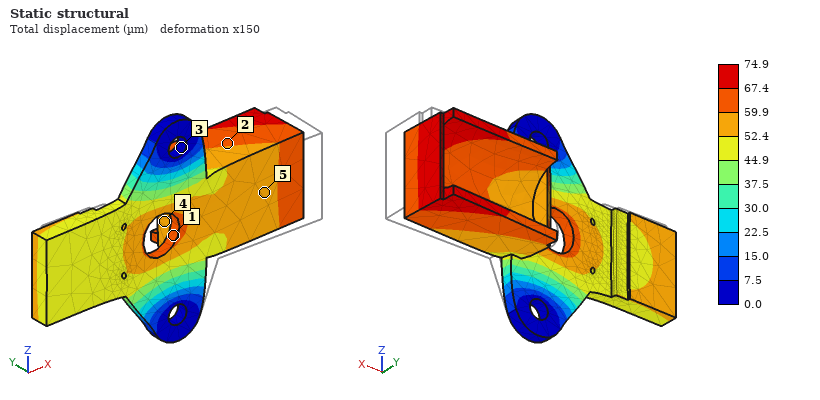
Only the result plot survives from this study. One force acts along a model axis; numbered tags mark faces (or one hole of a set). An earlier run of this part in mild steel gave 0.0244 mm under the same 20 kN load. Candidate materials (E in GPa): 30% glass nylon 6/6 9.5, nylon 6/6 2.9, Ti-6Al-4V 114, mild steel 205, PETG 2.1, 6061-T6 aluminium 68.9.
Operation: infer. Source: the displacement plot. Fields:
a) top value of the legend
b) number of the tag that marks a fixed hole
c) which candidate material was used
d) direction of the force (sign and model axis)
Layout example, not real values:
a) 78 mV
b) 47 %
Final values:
a) 74.9 µm
b) 3
c) 6061-T6 aluminium
d) -X
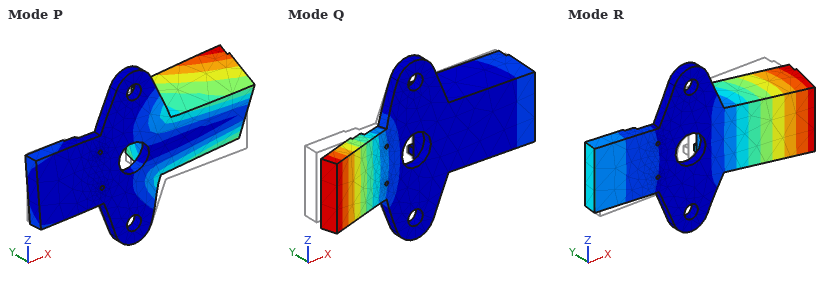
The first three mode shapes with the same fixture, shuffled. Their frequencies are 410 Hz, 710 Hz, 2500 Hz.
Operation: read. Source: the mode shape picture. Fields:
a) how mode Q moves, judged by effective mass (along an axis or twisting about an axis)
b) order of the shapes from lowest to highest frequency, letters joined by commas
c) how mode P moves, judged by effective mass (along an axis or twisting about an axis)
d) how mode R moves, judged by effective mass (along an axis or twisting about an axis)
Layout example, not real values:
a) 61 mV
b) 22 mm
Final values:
a) along Y
b) R, Q, P
c) along Z
d) along Y
